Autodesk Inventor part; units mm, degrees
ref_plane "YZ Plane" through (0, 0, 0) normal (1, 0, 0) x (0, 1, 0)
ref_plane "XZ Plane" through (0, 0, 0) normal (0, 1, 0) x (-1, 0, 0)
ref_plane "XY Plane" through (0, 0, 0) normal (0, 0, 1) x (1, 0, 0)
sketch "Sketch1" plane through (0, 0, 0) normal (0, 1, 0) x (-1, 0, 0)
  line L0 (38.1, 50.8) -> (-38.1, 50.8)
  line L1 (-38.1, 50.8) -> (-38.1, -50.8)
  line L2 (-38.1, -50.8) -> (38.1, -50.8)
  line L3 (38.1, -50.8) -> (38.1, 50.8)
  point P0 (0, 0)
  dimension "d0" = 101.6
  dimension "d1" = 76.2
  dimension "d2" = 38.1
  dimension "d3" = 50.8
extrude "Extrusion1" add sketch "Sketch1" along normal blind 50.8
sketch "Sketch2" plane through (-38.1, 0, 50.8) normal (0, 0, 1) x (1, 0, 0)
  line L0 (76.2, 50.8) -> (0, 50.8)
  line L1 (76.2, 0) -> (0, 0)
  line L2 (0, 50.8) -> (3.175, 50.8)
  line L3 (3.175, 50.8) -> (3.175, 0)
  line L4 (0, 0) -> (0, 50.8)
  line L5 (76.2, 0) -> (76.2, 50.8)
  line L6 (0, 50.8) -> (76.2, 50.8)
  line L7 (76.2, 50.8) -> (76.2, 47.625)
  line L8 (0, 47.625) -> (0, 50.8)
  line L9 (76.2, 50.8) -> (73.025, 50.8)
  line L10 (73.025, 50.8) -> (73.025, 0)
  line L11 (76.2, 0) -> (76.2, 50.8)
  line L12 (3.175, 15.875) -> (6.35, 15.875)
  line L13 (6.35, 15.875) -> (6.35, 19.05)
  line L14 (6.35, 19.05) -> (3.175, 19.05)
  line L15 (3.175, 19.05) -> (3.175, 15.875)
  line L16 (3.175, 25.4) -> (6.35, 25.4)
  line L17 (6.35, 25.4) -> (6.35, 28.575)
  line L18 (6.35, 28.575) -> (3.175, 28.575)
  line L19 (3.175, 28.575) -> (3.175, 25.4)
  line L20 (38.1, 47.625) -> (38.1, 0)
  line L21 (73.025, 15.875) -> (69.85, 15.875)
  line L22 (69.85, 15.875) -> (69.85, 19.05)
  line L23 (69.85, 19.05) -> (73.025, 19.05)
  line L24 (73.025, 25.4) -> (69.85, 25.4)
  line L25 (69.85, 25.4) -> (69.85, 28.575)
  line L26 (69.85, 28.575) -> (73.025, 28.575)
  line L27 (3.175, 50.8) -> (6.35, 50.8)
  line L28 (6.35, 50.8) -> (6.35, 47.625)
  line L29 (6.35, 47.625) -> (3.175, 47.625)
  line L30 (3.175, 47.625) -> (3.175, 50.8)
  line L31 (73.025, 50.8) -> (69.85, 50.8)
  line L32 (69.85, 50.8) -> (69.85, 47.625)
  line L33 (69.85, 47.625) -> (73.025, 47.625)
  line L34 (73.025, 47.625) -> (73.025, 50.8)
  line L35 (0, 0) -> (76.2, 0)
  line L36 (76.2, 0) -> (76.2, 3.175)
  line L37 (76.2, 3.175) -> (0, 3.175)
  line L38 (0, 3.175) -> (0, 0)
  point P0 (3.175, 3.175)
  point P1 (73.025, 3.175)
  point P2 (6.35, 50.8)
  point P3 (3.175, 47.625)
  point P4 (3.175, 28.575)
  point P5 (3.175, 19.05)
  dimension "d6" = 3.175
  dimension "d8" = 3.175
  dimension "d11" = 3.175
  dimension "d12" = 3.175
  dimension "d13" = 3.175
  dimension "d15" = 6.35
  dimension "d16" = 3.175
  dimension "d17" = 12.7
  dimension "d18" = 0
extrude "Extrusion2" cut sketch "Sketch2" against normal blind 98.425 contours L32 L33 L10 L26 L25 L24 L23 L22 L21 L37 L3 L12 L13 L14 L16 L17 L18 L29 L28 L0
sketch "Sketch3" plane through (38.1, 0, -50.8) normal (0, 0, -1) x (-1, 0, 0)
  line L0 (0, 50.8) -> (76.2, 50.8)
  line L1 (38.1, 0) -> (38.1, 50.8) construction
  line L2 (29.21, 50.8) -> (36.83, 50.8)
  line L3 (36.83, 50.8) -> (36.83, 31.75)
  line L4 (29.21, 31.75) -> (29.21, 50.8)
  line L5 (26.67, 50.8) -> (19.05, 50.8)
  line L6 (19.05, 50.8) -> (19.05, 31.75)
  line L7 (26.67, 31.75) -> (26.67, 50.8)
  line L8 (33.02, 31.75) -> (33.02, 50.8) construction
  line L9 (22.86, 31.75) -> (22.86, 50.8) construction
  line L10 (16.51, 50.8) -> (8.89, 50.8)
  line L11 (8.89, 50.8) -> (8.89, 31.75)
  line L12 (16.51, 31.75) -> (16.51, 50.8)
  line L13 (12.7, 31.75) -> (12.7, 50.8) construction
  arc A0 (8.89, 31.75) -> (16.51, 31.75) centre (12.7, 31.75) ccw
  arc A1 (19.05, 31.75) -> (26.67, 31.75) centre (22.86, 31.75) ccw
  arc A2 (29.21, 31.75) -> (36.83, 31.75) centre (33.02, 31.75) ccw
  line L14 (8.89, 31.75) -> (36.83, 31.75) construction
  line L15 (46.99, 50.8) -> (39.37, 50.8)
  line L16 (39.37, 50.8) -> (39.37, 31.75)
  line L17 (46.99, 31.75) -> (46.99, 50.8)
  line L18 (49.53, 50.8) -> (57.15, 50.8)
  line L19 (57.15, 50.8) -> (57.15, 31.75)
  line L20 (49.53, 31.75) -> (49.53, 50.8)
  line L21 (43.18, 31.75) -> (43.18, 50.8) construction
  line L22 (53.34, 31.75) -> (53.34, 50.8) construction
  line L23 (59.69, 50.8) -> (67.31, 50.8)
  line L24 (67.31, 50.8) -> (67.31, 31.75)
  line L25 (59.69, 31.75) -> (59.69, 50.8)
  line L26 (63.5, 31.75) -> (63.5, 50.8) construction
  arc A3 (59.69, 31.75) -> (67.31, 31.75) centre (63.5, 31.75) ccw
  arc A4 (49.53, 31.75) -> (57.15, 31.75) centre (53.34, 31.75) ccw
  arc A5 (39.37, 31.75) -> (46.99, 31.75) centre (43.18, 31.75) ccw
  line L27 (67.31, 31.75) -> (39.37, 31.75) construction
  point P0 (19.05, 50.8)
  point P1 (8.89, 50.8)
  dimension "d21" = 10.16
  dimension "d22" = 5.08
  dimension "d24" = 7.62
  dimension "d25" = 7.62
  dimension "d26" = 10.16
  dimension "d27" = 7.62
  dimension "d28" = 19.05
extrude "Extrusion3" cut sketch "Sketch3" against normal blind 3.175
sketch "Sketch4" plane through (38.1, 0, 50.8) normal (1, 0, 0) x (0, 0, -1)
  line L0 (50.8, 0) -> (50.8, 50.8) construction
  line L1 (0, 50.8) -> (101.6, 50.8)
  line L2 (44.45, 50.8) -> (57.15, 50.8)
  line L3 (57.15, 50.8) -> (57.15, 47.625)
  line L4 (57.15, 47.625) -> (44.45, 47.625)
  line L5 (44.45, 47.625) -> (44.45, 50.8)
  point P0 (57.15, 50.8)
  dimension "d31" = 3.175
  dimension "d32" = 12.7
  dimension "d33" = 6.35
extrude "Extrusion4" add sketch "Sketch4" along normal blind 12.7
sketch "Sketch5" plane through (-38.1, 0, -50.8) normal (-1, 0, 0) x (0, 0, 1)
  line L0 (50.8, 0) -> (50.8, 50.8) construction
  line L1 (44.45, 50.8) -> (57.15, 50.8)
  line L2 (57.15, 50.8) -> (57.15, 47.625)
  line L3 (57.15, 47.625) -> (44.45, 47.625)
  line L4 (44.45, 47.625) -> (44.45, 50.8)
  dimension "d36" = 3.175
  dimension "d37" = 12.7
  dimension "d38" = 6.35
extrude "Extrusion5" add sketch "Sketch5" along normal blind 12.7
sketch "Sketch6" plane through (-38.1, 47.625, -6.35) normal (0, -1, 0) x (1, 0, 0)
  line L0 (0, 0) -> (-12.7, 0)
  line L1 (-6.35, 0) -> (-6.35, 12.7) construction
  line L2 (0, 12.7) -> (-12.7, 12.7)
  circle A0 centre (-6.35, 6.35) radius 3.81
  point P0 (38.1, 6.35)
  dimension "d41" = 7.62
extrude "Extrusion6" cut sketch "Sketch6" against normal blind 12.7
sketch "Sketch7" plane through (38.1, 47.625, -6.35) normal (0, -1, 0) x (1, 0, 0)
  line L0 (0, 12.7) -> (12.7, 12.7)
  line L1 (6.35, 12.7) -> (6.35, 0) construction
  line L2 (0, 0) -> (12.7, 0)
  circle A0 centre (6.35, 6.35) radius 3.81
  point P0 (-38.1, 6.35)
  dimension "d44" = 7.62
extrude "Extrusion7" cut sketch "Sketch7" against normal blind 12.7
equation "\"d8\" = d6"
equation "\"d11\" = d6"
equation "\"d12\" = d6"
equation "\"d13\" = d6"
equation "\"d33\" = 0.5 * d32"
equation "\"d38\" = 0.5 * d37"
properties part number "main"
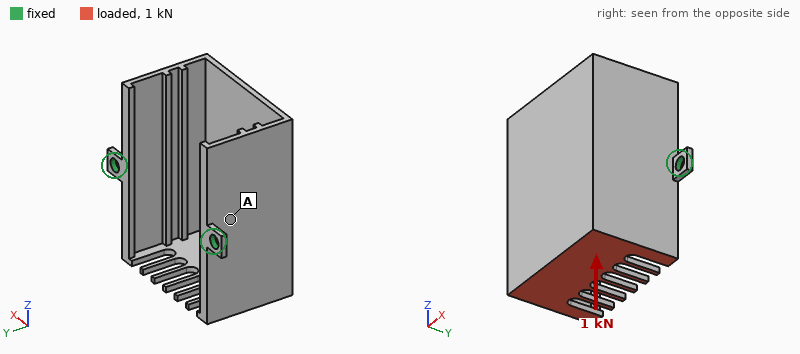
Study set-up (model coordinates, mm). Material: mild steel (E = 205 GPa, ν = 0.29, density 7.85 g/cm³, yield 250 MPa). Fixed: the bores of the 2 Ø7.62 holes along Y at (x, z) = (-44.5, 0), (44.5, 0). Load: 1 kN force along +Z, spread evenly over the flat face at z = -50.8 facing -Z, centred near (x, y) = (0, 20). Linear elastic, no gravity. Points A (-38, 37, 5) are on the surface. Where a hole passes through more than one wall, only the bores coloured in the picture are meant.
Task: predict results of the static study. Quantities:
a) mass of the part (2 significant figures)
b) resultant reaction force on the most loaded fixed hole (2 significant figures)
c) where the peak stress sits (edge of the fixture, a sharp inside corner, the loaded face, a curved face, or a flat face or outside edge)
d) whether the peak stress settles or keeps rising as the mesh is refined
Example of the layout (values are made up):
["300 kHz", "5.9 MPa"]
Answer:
["540 g", "500 N", "edge of the fixture", "keeps rising"]
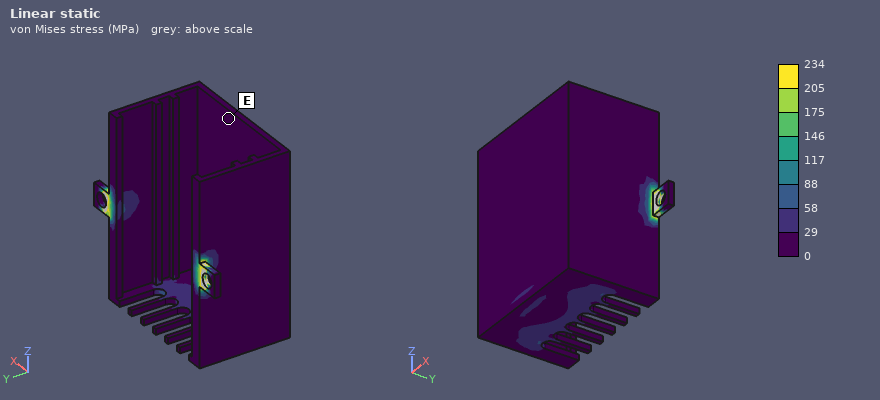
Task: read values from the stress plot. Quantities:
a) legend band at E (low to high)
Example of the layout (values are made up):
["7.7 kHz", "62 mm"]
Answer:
["0 to 29 MPa"]
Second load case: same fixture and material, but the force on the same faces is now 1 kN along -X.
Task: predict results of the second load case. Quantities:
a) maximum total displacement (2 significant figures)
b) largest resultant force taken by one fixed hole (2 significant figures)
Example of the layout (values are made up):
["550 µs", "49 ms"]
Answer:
["0.31 mm", "700 N"]
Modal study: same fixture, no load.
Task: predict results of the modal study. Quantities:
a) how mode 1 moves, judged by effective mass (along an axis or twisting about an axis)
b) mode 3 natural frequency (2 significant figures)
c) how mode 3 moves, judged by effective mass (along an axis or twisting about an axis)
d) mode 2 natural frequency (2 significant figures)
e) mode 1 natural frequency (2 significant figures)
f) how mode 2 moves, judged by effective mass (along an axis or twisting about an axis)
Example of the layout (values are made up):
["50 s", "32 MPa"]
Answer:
["along Z", "790 Hz", "along X", "590 Hz", "390 Hz", "along X"]
